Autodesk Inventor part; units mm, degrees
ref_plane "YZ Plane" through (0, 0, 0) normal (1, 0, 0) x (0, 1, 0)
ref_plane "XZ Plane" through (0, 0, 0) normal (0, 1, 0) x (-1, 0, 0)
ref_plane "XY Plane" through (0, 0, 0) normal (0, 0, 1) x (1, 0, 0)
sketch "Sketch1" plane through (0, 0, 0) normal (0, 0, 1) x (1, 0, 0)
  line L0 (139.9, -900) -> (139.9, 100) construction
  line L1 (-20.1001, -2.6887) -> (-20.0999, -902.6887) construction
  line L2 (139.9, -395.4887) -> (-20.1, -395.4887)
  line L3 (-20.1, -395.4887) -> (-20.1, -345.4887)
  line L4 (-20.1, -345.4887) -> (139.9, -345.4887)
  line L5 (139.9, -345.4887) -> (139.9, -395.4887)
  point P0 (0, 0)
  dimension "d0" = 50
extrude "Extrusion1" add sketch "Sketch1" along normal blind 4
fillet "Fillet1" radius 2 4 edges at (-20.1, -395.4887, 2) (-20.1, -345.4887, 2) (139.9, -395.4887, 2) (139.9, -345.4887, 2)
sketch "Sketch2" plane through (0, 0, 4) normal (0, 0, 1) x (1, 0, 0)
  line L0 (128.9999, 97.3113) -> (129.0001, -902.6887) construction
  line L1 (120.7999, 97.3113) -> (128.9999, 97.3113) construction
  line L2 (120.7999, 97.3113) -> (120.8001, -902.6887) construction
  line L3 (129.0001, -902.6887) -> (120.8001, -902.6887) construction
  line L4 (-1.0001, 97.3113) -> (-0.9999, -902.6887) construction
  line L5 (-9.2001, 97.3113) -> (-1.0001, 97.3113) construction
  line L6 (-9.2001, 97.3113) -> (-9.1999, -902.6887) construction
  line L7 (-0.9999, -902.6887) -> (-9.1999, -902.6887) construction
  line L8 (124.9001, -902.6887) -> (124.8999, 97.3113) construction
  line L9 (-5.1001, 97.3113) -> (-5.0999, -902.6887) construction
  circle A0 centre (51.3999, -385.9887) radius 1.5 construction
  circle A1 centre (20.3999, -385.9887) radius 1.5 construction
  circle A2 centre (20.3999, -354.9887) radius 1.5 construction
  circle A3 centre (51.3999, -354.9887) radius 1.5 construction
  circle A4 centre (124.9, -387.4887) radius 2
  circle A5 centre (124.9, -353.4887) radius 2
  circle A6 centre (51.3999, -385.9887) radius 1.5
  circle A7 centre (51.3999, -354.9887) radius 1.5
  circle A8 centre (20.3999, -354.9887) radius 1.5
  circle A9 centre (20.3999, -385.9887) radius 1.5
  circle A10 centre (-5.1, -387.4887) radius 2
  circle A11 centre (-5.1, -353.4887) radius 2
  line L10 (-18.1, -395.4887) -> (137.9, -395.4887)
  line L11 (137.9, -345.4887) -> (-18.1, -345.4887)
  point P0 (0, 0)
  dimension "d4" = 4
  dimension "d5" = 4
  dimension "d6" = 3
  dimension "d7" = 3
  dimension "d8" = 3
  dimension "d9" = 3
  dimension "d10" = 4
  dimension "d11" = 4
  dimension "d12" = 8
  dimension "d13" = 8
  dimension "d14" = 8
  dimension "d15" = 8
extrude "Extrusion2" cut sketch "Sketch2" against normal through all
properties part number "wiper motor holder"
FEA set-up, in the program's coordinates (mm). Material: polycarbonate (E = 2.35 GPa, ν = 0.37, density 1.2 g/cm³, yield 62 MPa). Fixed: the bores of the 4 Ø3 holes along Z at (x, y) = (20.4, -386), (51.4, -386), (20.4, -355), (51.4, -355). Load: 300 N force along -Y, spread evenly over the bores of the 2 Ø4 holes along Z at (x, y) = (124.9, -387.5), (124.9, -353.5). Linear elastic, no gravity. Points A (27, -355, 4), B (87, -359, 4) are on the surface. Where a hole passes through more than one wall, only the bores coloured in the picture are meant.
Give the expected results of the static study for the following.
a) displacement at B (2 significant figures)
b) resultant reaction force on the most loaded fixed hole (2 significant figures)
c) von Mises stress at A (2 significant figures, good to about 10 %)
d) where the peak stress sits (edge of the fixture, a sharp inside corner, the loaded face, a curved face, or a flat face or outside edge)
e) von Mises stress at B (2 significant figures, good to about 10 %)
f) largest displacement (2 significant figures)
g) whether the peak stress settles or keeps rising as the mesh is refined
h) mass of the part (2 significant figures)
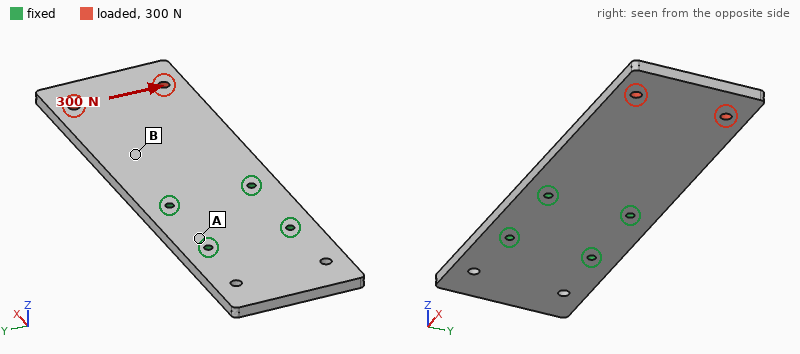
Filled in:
0.26 mm
560 N
1.9 MPa
edge of the fixture
4.4 MPa
0.83 mm
keeps rising
38 g
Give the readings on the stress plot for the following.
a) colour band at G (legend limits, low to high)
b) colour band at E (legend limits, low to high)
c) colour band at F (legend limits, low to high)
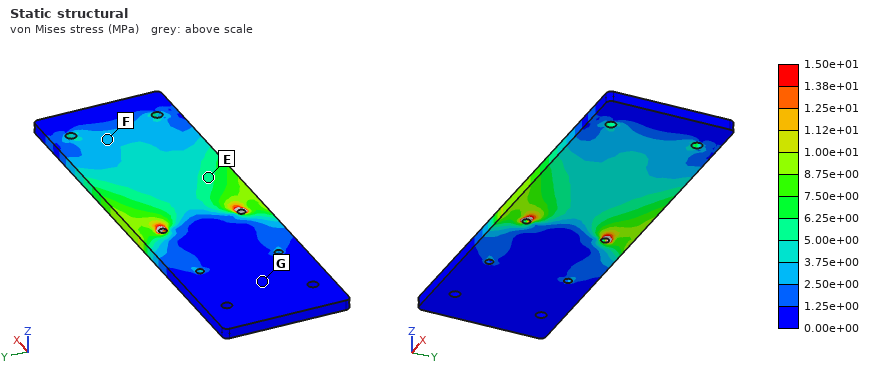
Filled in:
0.00e+00 to 1.25e+00 MPa
5.00e+00 to 6.25e+00 MPa
2.50e+00 to 3.75e+00 MPa
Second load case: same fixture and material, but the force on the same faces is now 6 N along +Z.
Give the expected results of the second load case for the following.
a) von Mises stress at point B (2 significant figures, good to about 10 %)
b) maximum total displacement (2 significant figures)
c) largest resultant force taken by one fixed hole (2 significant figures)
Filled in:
1.6 MPa
1.7 mm
5.4 N
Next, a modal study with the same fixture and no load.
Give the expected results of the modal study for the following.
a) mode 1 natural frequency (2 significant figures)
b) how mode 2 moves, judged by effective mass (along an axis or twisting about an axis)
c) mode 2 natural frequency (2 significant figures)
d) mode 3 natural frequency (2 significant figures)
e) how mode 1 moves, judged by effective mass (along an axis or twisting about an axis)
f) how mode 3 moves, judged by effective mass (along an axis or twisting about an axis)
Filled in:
110 Hz
twisting about X
430 Hz
530 Hz
along Z
along Z
